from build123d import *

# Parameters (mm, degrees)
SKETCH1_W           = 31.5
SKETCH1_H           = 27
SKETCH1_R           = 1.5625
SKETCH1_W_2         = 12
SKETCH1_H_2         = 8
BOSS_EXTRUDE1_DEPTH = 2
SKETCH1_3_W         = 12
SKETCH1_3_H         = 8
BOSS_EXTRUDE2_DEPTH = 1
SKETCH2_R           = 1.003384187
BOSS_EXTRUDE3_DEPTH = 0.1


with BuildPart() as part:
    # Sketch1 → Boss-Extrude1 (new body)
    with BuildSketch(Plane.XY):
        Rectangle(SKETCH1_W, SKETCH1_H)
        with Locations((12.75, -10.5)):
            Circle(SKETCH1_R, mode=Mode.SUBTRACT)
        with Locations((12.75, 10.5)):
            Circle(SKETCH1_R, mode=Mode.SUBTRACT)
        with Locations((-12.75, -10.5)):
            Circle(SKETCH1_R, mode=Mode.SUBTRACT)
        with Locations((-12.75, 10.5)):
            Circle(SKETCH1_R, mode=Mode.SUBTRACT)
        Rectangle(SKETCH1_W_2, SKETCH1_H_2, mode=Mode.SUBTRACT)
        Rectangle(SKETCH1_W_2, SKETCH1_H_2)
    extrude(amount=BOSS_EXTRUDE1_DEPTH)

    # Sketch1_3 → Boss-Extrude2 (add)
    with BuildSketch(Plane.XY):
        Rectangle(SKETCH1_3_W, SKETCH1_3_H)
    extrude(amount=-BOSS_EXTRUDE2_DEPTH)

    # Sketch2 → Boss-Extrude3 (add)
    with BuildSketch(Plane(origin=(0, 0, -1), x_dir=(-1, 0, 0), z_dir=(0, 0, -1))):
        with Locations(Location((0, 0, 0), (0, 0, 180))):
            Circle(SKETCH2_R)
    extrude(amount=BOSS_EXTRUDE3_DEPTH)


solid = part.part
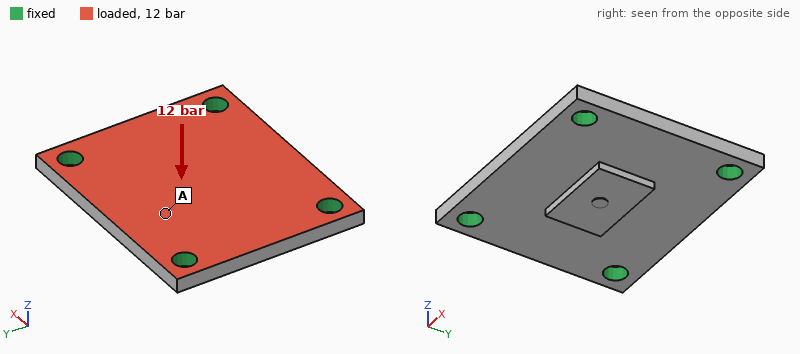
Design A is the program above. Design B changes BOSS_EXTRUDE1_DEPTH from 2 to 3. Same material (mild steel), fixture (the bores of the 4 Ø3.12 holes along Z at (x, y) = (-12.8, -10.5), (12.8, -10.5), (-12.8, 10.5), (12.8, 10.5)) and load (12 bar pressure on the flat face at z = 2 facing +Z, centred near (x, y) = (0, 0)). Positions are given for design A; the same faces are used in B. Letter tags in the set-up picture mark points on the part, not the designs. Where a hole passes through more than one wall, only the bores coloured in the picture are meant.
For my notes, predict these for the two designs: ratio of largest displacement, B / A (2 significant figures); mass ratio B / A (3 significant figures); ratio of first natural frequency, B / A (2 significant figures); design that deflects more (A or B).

0.37
1.47
1.4
A
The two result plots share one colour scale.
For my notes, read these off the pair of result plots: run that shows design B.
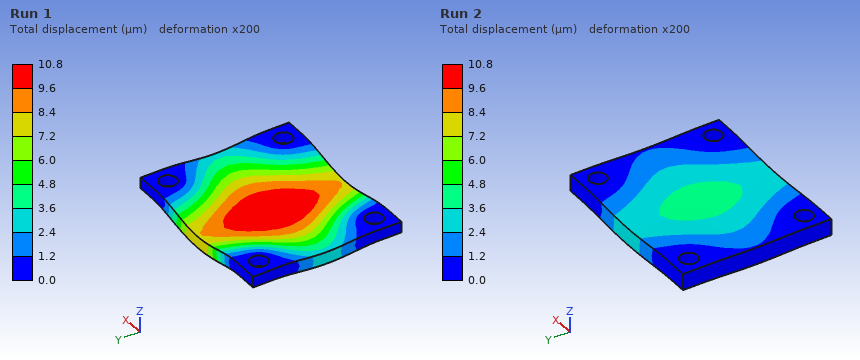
Run 2
